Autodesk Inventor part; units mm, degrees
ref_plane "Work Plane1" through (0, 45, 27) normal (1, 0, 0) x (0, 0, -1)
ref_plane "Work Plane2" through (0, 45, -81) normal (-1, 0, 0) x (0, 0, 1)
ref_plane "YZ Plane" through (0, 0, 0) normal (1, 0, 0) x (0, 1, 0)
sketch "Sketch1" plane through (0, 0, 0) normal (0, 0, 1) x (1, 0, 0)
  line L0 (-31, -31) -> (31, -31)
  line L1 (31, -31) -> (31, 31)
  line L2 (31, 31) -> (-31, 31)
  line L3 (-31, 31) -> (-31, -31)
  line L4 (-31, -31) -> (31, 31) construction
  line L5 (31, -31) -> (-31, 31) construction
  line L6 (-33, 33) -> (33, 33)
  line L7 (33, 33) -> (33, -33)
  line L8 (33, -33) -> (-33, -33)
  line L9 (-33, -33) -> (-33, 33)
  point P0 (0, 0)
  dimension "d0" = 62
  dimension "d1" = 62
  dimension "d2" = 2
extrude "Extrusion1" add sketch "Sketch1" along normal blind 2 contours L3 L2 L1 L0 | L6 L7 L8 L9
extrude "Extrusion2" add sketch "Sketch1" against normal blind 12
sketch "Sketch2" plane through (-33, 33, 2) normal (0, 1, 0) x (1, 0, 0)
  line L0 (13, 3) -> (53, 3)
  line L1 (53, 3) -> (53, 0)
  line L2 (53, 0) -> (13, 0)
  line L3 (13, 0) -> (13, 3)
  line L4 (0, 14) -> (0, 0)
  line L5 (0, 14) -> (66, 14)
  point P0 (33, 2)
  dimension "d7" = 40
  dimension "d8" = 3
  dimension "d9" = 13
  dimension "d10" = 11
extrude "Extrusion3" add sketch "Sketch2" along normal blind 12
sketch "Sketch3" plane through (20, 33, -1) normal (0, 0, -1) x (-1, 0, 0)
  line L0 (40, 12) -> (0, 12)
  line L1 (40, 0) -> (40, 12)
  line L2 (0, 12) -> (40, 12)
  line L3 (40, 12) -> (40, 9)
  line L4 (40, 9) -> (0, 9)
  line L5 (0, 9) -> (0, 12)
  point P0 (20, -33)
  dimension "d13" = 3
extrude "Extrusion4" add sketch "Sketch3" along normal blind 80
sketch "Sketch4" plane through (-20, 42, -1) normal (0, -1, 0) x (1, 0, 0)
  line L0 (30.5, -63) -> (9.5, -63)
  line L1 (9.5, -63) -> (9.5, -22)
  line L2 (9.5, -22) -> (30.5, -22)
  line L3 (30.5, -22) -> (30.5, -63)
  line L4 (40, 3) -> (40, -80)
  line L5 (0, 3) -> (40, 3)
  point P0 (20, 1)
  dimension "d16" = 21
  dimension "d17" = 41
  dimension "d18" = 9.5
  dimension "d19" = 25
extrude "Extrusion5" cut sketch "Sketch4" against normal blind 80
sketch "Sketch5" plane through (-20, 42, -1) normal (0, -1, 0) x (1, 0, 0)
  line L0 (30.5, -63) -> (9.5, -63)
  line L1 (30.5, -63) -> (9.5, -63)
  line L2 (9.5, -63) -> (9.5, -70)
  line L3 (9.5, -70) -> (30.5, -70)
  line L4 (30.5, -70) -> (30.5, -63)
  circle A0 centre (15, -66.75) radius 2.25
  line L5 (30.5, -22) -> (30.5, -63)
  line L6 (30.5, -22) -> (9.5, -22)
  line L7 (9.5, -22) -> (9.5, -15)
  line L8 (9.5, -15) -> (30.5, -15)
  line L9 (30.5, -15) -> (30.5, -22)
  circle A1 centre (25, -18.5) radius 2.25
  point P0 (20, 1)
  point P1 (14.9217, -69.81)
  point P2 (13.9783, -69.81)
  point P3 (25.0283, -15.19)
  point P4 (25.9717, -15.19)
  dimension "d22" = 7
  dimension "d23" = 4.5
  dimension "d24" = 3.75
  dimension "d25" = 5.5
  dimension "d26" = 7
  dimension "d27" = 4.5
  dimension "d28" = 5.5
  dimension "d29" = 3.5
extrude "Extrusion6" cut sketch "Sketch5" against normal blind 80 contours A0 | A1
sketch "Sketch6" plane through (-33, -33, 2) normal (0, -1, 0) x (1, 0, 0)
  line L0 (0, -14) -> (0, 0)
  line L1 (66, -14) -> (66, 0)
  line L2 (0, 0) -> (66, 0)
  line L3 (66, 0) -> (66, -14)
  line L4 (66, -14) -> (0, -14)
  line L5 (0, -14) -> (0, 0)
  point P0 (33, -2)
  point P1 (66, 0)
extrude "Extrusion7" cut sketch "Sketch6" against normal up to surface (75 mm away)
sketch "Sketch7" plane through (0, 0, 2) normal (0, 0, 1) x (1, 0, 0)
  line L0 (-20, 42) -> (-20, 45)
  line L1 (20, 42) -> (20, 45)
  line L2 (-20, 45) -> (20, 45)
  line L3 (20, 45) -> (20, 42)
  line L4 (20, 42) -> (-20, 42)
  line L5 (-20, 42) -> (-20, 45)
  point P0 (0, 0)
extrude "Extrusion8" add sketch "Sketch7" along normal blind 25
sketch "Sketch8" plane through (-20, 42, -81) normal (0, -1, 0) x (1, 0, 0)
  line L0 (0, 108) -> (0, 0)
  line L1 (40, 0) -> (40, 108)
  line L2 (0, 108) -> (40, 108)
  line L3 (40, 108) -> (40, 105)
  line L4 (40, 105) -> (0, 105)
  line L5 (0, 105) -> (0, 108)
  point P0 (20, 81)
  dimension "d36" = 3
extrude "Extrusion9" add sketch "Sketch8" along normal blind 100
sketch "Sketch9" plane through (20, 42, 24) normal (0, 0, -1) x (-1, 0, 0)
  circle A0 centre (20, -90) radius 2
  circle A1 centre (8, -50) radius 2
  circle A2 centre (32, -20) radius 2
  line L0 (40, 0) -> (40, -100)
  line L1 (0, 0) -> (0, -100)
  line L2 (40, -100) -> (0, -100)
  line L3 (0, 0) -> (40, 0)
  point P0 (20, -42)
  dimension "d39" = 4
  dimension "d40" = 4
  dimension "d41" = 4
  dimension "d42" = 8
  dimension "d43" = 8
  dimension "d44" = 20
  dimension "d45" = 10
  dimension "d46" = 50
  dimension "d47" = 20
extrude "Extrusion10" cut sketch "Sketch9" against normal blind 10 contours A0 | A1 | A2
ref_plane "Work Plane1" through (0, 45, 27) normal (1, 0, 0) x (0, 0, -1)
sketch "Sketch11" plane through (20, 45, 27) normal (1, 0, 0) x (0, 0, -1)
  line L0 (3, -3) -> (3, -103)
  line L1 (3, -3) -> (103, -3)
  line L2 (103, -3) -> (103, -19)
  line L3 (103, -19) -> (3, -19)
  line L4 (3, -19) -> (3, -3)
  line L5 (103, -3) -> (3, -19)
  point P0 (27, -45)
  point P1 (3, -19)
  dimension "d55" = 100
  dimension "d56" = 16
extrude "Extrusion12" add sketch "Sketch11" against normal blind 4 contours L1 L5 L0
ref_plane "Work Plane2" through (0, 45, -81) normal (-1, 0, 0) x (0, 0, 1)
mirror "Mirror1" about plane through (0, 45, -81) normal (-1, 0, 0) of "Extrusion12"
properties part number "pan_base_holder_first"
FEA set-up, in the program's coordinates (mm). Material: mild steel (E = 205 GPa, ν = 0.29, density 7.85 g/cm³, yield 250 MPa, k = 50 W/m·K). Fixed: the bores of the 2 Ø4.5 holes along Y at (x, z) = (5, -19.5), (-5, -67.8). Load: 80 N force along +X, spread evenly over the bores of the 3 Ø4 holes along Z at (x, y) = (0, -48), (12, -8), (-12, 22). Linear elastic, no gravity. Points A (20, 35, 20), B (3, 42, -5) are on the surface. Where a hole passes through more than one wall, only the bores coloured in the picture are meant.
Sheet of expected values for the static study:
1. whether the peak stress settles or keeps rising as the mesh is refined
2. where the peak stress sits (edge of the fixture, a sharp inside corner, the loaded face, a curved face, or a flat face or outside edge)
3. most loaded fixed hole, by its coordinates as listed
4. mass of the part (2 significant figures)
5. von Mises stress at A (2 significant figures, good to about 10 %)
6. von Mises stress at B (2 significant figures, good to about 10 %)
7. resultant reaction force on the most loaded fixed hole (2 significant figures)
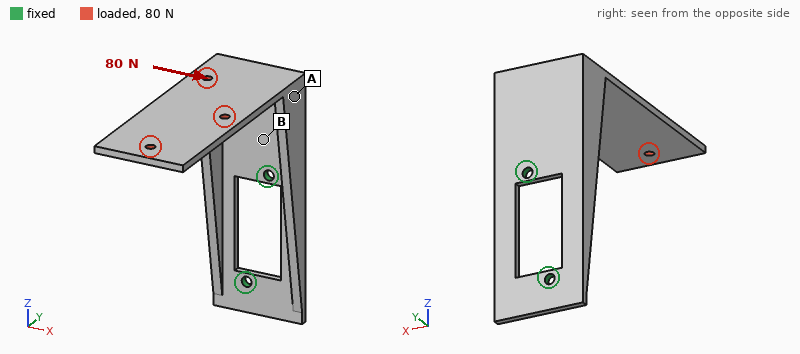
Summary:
keeps rising
edge of the fixture
(5, -19.5)
220 g
14 MPa
31 MPa
130 N
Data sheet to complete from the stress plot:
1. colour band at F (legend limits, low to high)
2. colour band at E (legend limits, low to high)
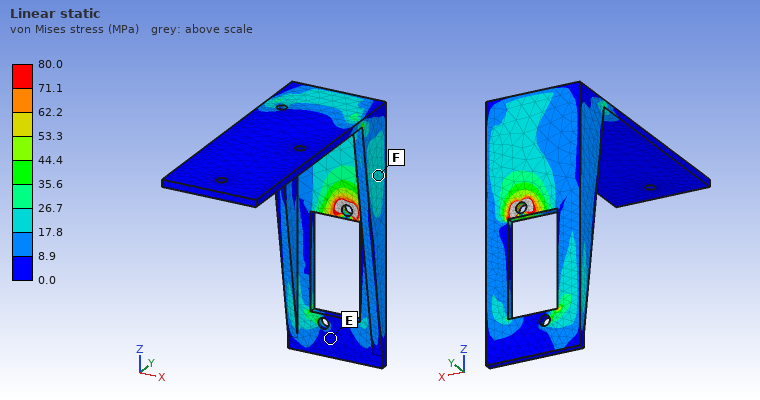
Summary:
17.8 to 26.7 MPa
0.0 to 8.9 MPa
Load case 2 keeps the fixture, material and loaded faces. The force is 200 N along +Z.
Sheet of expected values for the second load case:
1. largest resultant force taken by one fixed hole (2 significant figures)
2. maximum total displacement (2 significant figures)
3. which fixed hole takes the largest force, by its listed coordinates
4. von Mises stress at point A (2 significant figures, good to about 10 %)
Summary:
370 N
1.1 mm
(-5, -67.8)
26 MPa
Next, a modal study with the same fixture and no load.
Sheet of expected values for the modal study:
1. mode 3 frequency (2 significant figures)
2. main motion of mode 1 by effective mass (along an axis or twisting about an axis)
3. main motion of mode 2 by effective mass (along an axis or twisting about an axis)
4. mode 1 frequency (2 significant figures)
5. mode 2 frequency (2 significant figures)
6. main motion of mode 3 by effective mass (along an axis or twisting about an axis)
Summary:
850 Hz
along Z
along X
280 Hz
310 Hz
along Y
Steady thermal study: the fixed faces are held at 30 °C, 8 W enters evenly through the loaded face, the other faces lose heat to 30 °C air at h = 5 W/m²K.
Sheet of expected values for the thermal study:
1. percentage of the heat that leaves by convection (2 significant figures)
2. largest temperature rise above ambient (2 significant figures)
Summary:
39 %
76 K
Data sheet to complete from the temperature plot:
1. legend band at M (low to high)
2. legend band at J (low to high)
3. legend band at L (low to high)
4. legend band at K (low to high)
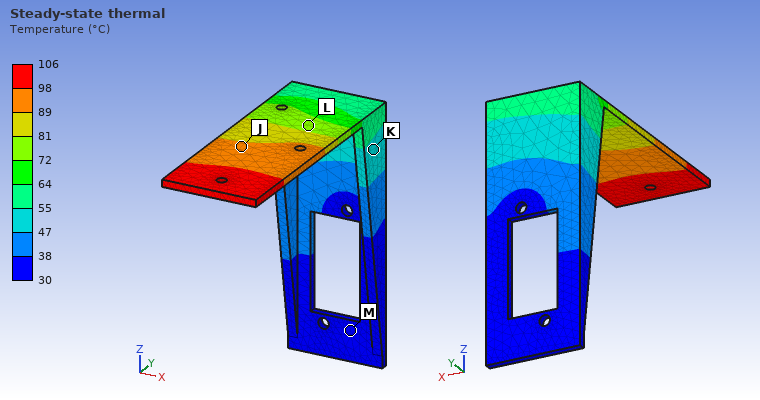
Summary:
30 to 38 °C
89 to 98 °C
72 to 81 °C
47 to 55 °C
